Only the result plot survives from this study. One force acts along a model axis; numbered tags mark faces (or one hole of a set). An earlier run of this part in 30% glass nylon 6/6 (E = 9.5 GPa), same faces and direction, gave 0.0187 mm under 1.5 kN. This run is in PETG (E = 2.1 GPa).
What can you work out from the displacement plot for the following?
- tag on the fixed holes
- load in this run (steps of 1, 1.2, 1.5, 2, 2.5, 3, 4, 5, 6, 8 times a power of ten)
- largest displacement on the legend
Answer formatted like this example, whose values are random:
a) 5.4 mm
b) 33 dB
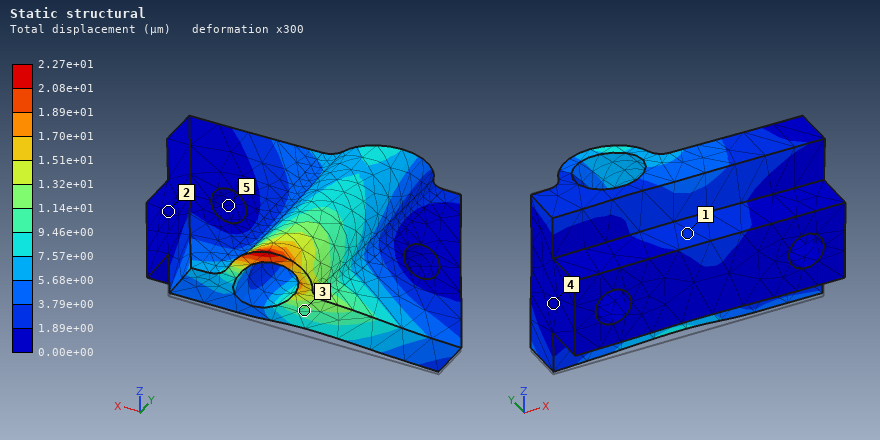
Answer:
a) 5
b) 400 N
c) 2.27e+01 µm
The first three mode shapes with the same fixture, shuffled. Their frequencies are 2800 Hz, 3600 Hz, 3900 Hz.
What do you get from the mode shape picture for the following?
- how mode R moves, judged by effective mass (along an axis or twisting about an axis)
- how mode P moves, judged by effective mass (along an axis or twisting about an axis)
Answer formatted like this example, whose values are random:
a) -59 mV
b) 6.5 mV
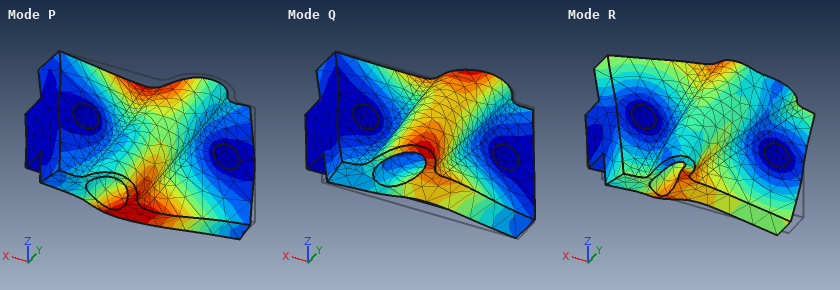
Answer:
a) along Z
b) along Y
